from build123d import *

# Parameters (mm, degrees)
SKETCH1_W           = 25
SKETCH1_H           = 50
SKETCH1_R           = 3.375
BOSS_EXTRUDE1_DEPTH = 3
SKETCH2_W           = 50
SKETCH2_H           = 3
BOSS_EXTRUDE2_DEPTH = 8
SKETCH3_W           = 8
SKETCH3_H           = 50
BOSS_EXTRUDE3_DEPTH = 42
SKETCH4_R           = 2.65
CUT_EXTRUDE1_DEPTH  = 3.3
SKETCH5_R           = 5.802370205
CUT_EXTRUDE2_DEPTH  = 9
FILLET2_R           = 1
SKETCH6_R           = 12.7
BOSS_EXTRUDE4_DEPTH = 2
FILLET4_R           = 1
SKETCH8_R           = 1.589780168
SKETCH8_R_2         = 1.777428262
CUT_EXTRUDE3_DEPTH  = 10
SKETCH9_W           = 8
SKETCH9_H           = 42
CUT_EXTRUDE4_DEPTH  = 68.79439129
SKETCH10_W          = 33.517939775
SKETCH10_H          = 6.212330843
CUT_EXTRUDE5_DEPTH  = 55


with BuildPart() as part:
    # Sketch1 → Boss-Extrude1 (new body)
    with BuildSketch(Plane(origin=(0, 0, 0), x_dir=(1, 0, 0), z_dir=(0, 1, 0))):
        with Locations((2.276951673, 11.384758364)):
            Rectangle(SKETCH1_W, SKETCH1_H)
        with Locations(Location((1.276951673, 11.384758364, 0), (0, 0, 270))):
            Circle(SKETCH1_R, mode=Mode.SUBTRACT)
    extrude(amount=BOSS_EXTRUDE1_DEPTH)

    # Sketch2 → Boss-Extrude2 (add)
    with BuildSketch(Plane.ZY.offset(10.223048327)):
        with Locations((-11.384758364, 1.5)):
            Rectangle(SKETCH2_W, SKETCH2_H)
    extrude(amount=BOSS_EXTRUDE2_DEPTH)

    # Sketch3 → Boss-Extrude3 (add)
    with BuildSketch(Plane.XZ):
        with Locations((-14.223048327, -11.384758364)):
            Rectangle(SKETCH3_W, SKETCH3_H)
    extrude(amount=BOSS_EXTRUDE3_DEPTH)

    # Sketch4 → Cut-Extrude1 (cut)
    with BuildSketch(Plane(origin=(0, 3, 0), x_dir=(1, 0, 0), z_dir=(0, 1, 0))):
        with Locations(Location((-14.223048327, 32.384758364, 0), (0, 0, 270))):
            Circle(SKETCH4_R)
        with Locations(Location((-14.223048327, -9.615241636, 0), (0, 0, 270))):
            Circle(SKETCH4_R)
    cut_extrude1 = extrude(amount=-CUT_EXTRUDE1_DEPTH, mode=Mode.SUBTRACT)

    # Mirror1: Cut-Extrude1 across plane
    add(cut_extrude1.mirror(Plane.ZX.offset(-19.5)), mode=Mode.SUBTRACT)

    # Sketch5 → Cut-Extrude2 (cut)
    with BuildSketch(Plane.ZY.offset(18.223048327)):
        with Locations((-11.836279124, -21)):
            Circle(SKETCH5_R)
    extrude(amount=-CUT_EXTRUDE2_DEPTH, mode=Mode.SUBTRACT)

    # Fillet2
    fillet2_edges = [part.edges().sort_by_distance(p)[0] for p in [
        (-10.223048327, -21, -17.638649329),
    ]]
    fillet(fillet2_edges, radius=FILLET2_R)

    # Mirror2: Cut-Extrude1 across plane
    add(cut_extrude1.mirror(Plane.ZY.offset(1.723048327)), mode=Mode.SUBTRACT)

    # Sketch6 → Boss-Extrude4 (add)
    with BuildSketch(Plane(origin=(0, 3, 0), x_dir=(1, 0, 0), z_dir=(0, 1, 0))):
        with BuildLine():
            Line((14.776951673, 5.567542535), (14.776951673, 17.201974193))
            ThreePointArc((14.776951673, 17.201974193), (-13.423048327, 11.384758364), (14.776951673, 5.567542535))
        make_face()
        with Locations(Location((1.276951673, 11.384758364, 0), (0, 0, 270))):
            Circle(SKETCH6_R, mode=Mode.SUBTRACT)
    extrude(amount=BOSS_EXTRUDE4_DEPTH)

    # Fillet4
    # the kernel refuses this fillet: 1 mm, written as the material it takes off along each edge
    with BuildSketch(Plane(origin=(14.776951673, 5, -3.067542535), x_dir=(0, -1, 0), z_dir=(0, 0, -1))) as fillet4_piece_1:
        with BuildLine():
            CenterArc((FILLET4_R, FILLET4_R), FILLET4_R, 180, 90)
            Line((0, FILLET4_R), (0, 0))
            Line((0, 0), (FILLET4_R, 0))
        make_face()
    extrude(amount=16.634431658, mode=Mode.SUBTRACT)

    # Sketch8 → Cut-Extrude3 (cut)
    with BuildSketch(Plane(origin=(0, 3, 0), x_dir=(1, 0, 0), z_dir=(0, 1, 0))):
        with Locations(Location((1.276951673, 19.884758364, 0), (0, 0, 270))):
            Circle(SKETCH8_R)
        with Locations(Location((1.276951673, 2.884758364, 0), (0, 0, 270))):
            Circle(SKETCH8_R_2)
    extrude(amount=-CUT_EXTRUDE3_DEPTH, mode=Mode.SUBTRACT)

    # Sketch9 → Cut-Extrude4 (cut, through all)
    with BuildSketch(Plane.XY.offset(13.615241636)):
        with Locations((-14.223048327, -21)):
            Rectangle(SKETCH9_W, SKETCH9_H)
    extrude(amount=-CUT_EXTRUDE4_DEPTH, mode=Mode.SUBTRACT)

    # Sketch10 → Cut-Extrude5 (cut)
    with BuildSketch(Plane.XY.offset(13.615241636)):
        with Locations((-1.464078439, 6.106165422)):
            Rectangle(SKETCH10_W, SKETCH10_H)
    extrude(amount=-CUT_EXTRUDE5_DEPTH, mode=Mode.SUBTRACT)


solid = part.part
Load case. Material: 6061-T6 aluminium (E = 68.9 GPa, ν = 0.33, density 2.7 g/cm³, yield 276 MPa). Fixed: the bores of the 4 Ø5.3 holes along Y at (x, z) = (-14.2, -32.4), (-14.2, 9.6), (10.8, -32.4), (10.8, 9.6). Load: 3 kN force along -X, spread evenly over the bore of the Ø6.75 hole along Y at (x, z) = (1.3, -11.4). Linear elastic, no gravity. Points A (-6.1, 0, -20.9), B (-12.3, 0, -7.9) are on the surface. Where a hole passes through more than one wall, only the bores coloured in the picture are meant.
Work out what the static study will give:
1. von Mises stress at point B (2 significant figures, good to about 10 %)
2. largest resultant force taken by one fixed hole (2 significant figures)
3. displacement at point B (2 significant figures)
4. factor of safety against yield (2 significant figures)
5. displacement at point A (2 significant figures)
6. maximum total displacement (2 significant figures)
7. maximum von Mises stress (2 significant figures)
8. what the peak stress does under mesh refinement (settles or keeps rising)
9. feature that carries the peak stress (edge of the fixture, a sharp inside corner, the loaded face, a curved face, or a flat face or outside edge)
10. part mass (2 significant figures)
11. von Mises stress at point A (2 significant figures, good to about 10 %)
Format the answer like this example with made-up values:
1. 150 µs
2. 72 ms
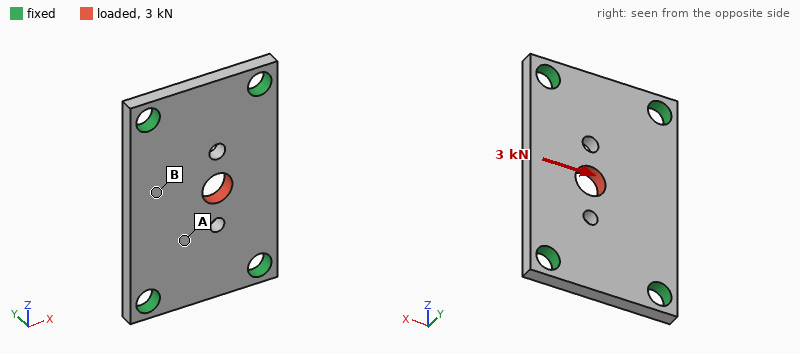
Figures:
1. 17 MPa
2. 990 N
3. 11 µm
4. 2.9
5. 8.1 µm
6. 18 µm
7. 94 MPa
8. settles
9. the loaded face
10. 12 g
11. 38 MPa
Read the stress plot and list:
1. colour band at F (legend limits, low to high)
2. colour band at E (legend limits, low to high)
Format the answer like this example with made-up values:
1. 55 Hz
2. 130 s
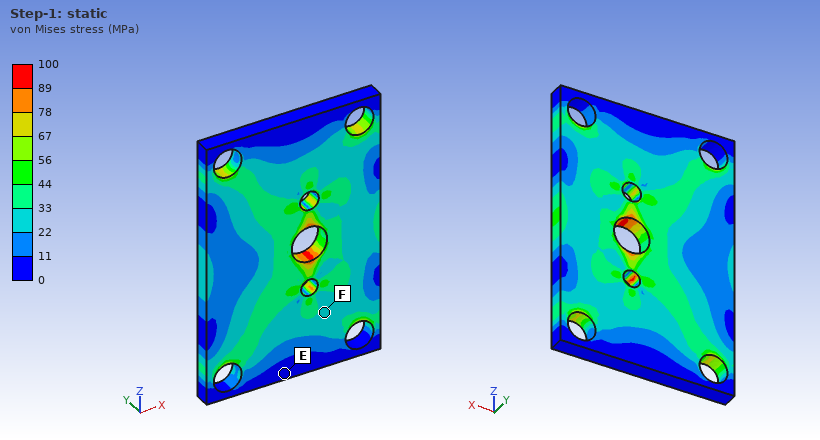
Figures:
1. 22 to 33 MPa
2. 0 to 11 MPa
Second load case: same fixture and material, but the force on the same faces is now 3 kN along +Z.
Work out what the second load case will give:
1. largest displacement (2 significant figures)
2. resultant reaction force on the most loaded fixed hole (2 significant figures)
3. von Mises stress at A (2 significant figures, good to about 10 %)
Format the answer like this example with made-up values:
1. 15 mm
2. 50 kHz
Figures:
1. 10 µm
2. 900 N
3. 22 MPa
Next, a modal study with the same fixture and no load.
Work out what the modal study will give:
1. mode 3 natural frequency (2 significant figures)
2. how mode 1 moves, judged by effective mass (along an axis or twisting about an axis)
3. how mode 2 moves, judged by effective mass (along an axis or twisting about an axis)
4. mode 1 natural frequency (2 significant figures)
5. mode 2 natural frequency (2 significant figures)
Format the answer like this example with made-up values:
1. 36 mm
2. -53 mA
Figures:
1. 20 kHz
2. along Y
3. twisting about Z
4. 9300 Hz
5. 13 kHz
